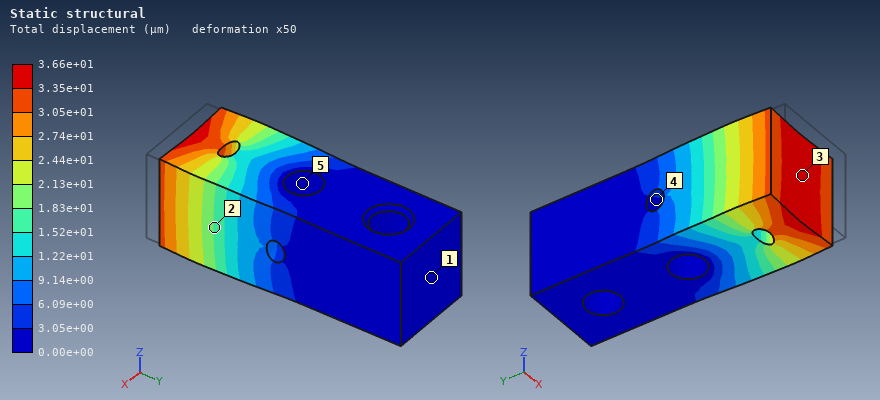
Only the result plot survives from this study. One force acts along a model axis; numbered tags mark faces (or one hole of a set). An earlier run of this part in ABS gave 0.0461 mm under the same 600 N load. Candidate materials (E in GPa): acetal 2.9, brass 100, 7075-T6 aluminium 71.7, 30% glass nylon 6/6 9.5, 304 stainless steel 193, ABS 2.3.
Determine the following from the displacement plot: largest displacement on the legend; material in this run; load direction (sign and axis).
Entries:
3.66e+01 µm
acetal
+Y
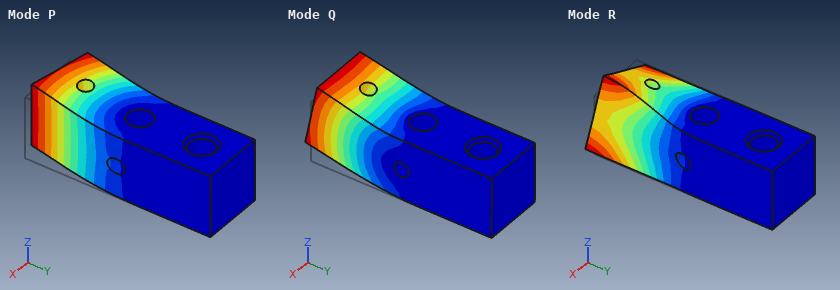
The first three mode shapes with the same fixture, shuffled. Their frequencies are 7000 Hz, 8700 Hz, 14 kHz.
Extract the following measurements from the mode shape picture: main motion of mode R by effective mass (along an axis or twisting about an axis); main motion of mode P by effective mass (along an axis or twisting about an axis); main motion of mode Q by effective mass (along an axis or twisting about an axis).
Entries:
twisting about Y
along X
along Z
